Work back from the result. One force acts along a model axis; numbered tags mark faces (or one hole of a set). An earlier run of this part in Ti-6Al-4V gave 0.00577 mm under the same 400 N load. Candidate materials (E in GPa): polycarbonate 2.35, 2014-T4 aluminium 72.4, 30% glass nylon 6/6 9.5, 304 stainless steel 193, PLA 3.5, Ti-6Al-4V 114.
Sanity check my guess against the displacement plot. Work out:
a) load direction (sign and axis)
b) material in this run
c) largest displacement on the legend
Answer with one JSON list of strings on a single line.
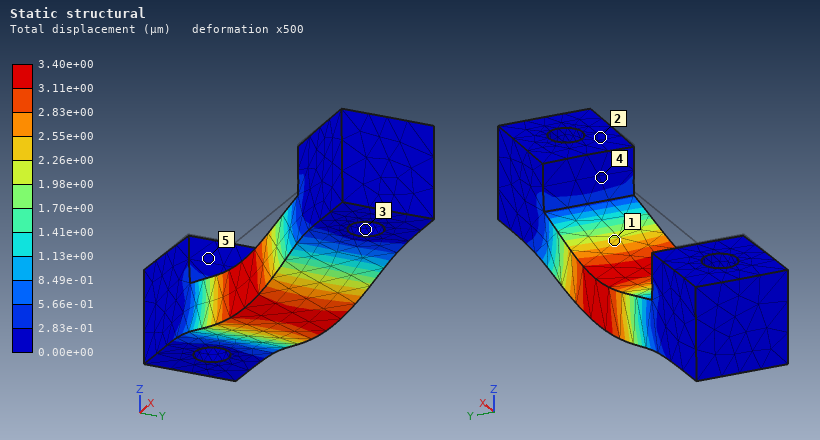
["-Z", "304 stainless steel", "3.40e+00 µm"]
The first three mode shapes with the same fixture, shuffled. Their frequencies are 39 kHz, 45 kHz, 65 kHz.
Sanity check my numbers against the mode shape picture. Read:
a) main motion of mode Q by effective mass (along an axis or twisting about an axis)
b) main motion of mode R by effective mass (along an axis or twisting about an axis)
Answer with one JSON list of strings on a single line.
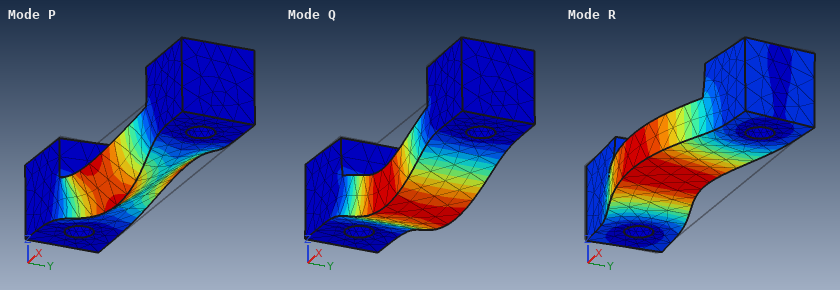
["along Z", "along Y"]
